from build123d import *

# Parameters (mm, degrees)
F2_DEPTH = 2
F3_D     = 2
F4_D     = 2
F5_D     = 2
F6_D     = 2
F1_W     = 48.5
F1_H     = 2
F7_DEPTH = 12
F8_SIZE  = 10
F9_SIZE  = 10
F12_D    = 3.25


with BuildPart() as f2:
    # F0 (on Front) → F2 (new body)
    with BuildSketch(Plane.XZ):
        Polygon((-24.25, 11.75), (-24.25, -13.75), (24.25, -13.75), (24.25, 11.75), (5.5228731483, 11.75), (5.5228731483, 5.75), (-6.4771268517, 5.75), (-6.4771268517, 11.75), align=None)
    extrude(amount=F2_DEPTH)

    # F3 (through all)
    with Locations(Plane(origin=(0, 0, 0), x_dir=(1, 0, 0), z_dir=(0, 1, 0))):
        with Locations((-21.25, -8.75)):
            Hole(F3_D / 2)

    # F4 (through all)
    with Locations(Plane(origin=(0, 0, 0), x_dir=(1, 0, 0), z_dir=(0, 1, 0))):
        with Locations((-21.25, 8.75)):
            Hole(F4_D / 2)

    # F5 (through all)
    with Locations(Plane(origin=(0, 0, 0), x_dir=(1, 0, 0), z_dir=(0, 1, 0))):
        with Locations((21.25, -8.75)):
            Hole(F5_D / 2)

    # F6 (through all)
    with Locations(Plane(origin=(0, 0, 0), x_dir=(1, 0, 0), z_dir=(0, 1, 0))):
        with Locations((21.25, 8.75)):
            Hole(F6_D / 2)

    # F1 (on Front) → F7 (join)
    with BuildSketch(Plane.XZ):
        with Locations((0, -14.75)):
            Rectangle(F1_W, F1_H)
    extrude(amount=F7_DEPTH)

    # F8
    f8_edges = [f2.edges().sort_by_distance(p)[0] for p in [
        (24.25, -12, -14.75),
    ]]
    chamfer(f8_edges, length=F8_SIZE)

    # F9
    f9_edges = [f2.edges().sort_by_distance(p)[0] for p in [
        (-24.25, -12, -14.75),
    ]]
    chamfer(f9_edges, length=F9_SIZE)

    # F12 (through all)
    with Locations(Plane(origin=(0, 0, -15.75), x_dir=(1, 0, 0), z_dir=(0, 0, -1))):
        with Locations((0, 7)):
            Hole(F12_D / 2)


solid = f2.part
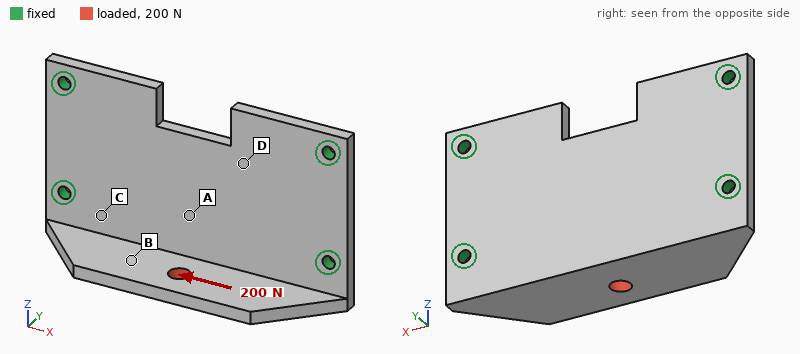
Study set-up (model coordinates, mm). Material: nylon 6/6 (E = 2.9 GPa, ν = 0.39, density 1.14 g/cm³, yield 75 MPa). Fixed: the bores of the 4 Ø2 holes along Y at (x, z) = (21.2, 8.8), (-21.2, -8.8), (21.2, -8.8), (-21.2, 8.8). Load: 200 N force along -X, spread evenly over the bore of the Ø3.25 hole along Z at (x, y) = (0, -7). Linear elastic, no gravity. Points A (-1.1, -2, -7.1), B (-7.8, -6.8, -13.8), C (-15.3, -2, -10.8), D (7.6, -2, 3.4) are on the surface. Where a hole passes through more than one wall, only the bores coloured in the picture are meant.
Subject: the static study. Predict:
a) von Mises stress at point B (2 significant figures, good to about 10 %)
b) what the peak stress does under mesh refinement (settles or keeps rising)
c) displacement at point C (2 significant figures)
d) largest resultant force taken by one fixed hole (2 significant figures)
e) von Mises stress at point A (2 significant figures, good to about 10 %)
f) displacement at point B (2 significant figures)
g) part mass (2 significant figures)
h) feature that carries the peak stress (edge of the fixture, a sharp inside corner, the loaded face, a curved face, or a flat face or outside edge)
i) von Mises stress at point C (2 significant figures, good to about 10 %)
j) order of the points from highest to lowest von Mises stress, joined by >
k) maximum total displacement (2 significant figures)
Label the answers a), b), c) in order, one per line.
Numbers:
a) 5.9 MPa
b) keeps rising
c) 0.029 mm
d) 92 N
e) 3.3 MPa
f) 0.074 mm
g) 3.7 g
h) edge of the fixture
i) 8.7 MPa
j) C > B > A > D
k) 0.14 mm
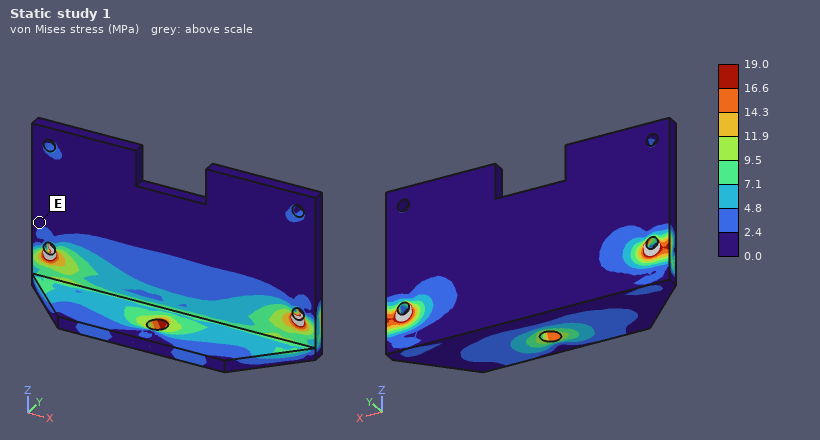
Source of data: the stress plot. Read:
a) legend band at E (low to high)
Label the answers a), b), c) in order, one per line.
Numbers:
a) 0.0 to 2.4 MPa
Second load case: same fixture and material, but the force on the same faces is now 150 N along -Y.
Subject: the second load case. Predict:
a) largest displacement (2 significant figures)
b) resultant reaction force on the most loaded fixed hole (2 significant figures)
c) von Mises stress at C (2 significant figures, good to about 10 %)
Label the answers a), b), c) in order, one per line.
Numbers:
a) 0.68 mm
b) 110 N
c) 16 MPa
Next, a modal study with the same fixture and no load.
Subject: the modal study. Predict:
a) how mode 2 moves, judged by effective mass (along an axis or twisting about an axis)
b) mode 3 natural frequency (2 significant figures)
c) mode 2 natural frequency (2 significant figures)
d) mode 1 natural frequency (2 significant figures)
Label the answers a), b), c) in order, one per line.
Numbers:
a) along Y
b) 3900 Hz
c) 2400 Hz
d) 2000 Hz
